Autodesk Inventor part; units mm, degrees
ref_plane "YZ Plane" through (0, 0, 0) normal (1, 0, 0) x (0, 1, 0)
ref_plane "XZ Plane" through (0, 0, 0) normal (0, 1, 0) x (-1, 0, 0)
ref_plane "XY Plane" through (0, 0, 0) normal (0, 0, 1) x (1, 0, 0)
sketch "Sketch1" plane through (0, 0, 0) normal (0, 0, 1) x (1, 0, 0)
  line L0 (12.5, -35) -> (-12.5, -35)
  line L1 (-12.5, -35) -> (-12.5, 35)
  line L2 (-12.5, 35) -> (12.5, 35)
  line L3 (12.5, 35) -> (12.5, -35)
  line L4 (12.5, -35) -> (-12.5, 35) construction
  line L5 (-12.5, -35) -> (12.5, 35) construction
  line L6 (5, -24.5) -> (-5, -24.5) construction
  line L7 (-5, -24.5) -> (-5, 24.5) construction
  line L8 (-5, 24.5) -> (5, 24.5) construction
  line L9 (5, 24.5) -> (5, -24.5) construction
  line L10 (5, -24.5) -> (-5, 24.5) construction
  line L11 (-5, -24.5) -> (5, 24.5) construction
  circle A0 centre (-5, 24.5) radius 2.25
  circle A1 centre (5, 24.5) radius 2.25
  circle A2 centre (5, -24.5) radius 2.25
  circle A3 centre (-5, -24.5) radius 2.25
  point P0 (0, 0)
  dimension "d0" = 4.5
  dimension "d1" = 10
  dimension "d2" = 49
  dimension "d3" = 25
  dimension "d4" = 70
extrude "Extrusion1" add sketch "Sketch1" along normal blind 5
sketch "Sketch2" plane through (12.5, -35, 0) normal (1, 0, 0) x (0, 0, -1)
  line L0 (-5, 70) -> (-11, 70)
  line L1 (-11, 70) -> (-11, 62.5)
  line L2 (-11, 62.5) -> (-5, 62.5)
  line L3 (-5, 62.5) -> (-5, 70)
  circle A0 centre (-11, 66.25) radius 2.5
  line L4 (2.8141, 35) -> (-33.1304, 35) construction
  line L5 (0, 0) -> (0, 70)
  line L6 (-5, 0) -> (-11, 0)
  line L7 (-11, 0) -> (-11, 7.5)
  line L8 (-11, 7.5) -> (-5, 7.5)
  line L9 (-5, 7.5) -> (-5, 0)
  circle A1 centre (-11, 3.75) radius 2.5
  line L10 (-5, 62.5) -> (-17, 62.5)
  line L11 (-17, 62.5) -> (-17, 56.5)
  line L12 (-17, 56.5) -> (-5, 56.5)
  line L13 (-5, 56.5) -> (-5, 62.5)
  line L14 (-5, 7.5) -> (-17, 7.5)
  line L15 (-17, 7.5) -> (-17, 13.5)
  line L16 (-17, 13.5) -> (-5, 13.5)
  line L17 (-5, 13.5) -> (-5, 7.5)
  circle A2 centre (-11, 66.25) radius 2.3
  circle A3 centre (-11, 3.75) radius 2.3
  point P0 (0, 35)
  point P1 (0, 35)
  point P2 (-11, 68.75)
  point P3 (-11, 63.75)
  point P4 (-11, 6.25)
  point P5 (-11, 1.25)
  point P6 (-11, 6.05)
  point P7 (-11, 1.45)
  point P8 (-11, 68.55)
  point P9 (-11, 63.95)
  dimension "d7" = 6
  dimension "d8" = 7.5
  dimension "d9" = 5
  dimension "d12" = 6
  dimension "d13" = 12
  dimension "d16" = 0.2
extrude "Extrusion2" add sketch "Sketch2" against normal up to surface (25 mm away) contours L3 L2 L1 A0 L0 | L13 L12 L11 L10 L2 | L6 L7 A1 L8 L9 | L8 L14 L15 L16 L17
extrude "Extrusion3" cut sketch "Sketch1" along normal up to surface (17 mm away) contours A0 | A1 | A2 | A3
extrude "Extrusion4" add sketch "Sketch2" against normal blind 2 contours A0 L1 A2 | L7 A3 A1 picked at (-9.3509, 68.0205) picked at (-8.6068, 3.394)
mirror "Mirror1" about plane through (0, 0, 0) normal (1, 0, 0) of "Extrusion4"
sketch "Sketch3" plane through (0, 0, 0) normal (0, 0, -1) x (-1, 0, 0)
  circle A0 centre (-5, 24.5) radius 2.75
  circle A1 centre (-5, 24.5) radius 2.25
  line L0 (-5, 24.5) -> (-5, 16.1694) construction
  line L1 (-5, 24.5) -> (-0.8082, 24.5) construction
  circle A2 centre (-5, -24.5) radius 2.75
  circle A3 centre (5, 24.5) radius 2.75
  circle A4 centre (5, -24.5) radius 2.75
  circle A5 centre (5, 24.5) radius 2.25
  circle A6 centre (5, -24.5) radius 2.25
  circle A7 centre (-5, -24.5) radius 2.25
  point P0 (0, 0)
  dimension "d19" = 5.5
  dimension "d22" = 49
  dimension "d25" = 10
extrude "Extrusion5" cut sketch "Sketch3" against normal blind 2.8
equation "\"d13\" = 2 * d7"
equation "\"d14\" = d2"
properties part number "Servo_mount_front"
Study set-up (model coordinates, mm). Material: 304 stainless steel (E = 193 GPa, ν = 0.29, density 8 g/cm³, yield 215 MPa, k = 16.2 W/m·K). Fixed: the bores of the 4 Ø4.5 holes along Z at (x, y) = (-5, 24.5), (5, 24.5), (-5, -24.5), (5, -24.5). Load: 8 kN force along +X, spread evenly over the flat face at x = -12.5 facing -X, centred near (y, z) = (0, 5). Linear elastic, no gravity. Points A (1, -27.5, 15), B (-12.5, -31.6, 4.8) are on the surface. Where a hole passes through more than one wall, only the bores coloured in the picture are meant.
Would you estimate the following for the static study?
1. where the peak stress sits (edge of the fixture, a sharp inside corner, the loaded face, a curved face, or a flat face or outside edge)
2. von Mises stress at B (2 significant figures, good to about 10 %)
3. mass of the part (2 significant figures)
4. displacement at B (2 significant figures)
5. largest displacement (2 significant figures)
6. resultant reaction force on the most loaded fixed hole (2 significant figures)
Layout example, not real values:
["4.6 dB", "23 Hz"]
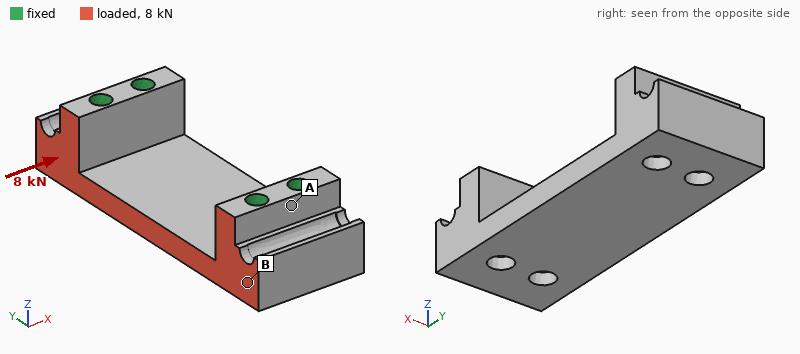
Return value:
["edge of the fixture", "16 MPa", "100 g", "1.1 µm", "4.4 µm", "2.9 kN"]
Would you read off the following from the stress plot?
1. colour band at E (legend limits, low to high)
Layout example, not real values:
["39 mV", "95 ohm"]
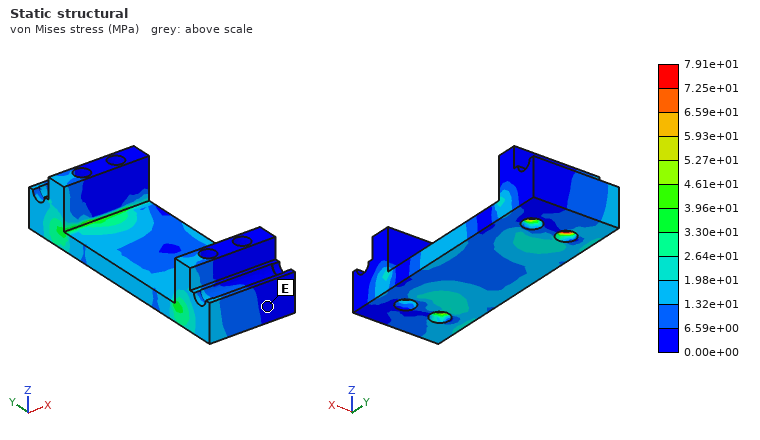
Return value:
["0.00e+00 to 6.59e+00 MPa"]
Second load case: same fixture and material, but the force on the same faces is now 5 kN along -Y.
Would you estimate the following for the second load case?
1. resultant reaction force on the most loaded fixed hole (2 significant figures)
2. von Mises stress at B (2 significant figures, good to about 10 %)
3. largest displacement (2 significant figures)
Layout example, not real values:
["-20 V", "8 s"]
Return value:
["2.4 kN", "20 MPa", "3.0 µm"]
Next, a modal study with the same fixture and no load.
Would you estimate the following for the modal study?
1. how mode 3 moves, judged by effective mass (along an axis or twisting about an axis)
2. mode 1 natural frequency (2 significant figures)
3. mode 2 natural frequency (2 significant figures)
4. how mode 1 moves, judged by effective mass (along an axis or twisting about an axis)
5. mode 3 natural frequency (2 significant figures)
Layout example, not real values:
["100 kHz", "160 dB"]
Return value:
["along X", "10 kHz", "15 kHz", "along Z", "23 kHz"]
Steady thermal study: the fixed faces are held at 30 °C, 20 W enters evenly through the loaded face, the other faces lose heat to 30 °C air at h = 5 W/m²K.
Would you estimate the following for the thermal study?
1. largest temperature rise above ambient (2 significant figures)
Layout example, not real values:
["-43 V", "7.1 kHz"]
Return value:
["45 K"]
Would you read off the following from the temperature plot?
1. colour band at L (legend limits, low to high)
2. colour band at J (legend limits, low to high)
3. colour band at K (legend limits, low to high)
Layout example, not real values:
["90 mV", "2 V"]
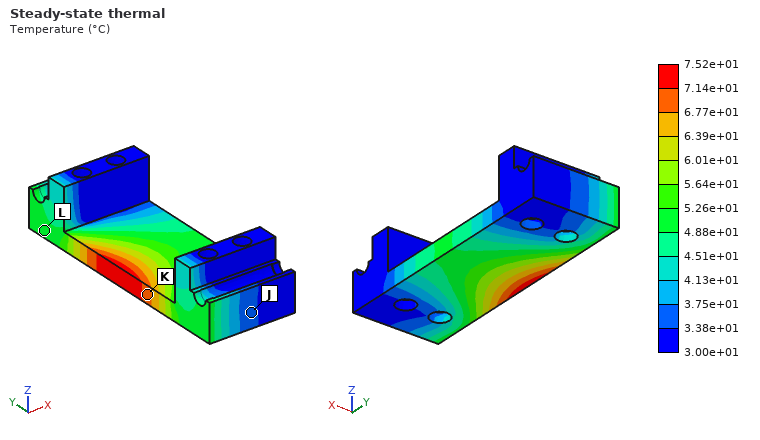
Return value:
["4.88e+01 to 5.26e+01 °C", "3.38e+01 to 3.75e+01 °C", "6.77e+01 to 7.14e+01 °C"]
